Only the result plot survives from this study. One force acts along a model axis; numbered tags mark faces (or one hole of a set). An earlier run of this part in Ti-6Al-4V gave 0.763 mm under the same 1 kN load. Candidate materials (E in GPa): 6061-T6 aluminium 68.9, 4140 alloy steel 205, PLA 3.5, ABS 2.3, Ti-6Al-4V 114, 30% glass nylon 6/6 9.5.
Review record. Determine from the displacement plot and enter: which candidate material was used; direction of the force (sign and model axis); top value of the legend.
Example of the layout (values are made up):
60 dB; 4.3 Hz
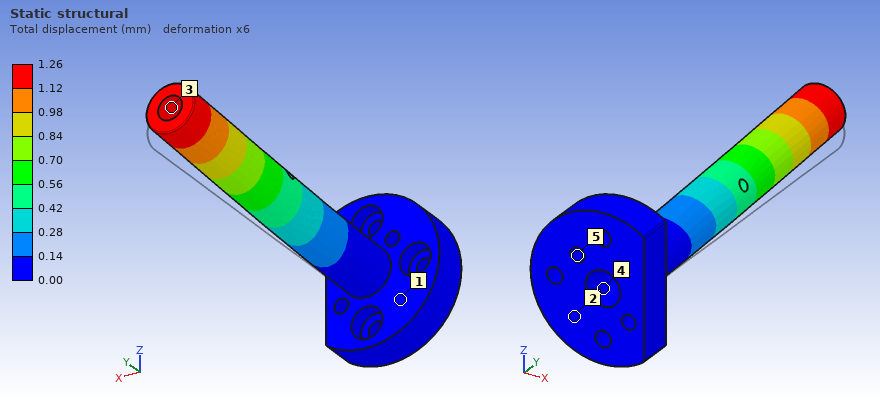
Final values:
6061-T6 aluminium; +Z; 1.26 mm
